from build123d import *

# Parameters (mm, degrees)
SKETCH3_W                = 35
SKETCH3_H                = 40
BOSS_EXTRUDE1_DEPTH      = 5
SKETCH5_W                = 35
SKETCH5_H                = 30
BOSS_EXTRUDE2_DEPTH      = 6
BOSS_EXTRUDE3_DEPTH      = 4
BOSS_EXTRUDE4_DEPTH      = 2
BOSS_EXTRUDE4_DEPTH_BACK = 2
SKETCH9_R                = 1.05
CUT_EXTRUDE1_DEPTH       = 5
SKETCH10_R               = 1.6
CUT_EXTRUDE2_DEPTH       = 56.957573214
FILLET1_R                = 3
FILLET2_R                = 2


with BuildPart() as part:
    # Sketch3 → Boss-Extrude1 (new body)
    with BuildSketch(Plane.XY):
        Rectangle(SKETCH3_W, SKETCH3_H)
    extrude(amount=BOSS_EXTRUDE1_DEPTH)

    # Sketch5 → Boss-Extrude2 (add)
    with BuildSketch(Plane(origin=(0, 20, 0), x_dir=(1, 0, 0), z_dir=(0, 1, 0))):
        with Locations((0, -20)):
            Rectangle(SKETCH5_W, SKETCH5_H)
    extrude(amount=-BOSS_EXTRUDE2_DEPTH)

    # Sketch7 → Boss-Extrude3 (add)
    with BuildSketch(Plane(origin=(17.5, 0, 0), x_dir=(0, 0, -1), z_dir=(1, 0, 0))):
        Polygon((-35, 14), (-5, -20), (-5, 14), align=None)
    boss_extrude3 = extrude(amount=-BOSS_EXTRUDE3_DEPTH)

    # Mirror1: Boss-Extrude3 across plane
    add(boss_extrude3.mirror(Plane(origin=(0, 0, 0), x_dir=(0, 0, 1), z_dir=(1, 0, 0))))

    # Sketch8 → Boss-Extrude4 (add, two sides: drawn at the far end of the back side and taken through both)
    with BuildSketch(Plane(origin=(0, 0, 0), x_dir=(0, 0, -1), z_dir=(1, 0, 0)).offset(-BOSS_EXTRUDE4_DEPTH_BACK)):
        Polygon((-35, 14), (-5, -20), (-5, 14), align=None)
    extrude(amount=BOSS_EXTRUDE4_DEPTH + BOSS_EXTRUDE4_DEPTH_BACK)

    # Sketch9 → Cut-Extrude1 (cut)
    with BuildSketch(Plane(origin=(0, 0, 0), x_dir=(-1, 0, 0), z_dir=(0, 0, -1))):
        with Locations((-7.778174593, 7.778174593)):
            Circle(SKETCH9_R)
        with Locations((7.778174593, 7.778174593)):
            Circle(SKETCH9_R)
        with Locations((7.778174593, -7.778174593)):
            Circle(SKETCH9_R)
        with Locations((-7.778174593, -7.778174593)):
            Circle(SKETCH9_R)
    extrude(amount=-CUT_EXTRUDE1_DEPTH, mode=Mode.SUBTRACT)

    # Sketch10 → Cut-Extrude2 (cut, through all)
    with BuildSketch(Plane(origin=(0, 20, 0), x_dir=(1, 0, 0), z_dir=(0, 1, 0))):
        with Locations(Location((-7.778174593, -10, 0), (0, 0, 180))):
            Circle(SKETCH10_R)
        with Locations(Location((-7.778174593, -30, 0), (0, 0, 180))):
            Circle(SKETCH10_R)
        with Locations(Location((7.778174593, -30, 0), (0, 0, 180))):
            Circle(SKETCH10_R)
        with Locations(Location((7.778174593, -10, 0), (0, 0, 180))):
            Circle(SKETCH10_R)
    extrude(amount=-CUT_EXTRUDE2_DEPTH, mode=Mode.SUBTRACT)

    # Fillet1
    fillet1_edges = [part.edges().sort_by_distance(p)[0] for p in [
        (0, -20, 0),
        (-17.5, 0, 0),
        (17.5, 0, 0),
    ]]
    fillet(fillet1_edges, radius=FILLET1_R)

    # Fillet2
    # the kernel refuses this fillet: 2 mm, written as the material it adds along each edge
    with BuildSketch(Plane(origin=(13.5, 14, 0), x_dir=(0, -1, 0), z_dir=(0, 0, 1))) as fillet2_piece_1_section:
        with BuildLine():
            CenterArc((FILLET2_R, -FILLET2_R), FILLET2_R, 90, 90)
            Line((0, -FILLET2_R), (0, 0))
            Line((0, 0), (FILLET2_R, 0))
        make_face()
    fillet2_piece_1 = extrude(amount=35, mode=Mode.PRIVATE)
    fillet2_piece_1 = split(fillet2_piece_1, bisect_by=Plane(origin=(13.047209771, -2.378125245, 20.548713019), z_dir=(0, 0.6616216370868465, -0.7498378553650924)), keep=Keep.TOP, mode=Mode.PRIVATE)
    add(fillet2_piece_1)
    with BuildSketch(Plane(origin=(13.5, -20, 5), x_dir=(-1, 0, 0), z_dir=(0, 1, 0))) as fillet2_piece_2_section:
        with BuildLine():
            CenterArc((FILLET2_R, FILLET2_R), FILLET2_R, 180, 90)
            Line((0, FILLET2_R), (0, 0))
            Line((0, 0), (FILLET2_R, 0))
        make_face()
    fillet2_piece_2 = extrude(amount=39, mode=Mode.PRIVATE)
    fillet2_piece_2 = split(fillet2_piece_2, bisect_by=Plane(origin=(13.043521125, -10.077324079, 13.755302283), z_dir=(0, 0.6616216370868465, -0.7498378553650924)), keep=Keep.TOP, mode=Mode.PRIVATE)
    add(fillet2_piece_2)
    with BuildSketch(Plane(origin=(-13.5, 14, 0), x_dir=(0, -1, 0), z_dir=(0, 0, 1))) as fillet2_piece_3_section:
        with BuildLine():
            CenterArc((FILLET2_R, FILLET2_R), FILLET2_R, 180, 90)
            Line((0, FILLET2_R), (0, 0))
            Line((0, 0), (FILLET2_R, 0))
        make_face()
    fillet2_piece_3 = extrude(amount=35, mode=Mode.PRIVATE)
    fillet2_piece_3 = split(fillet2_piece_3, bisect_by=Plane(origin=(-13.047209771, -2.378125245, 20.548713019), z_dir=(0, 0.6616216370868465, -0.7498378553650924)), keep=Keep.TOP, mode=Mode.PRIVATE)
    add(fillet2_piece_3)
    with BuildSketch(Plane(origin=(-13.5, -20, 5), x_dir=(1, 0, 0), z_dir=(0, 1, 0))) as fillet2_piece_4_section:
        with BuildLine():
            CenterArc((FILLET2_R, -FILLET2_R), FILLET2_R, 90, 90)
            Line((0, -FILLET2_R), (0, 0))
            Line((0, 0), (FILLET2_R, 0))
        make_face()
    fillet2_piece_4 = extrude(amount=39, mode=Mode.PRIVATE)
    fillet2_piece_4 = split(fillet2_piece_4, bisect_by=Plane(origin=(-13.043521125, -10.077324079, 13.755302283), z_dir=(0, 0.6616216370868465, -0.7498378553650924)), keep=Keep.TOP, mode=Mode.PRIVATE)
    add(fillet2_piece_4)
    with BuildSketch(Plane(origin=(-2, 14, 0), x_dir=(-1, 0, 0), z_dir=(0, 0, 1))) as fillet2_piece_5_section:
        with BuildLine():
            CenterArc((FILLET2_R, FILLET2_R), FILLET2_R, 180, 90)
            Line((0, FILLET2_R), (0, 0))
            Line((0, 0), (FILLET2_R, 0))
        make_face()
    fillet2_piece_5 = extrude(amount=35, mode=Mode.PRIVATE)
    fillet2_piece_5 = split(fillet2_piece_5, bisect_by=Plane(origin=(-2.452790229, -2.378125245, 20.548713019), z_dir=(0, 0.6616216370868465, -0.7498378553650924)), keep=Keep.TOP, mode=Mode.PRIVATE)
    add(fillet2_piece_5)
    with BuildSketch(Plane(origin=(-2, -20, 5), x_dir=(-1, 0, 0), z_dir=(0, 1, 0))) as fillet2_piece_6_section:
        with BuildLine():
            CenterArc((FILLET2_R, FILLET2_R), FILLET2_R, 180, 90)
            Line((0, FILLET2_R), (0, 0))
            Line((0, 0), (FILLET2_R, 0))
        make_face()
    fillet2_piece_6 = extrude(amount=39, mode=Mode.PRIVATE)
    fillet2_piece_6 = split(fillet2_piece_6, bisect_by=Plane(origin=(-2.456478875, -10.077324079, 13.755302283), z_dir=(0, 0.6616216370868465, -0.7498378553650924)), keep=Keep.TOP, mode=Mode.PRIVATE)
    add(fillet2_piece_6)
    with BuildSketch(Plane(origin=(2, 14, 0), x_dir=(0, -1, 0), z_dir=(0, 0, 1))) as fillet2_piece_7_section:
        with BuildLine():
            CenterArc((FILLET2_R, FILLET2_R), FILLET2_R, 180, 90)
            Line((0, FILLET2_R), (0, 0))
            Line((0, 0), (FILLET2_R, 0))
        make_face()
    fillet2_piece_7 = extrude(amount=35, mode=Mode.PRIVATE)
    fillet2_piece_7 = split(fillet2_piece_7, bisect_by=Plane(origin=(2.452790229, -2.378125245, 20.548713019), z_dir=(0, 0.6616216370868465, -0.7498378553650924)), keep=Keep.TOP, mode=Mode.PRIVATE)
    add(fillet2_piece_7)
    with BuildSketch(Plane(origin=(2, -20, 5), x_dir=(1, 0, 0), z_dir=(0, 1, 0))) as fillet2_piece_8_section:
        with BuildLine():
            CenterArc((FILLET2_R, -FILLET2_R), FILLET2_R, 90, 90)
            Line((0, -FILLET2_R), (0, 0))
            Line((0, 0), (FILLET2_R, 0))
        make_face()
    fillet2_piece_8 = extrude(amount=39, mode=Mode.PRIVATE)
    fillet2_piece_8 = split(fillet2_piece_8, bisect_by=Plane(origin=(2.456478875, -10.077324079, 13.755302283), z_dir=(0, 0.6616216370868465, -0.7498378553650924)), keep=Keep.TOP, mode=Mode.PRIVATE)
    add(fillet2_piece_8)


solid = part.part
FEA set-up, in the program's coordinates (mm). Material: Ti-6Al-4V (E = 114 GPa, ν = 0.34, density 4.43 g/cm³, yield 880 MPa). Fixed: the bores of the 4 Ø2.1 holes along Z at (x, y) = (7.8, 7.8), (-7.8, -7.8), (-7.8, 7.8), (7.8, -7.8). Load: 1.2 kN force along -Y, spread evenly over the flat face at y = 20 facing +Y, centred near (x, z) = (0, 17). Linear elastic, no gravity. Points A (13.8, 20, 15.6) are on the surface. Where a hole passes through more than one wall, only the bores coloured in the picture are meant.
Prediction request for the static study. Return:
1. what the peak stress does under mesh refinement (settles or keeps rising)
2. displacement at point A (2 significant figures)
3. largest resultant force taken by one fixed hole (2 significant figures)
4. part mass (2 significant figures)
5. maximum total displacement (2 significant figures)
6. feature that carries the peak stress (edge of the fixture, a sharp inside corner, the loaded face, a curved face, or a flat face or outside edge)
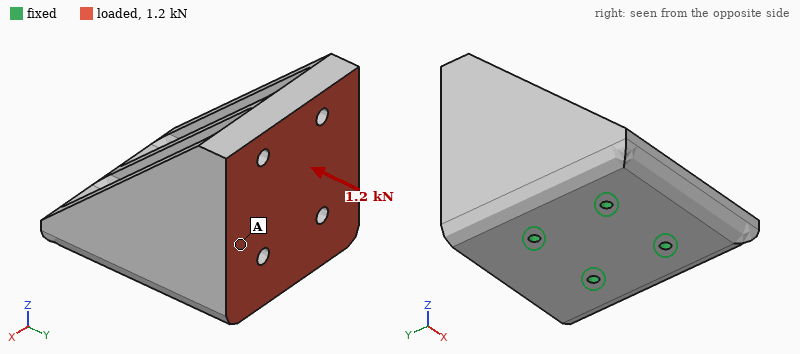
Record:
keeps rising
6.3 µm
550 N
85 g
11 µm
edge of the fixture
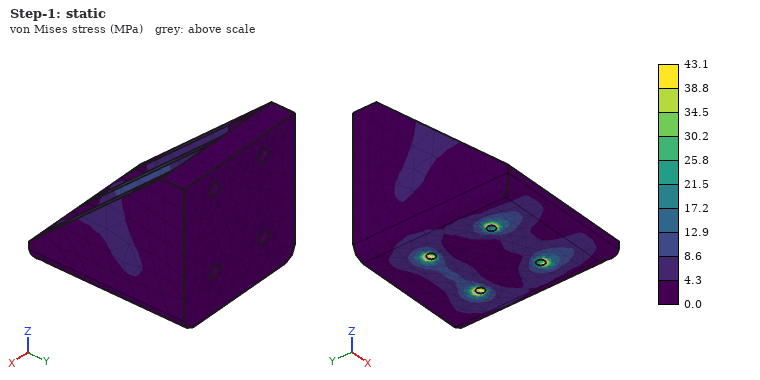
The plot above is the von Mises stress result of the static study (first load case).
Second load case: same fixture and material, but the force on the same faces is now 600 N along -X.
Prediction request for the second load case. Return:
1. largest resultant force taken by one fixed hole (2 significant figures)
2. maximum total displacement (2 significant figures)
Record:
550 N
9.6 µm
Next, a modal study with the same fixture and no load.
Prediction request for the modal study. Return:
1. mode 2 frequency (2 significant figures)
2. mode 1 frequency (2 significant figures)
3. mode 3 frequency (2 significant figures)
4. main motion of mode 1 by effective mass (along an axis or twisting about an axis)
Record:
8000 Hz
6100 Hz
13 kHz
along X
